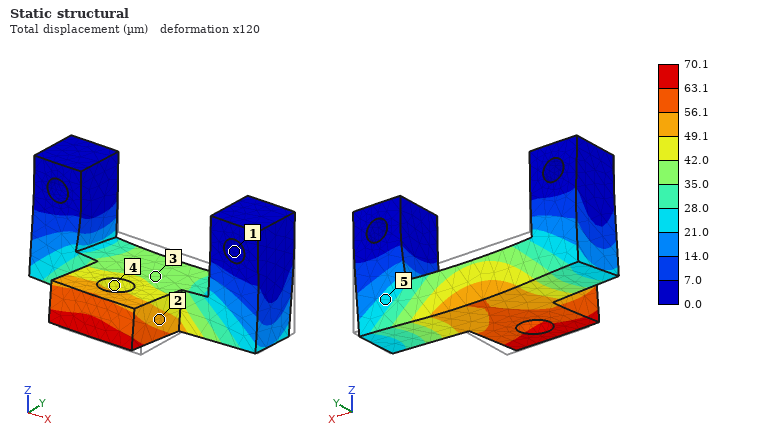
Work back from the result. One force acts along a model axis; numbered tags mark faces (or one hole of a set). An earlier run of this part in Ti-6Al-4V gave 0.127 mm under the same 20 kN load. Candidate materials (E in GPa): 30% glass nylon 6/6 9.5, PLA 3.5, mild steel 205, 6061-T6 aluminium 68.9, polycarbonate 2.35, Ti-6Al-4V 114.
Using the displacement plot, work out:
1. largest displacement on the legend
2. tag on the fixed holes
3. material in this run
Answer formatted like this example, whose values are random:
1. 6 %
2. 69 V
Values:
1. 70.1 µm
2. 1
3. mild steel
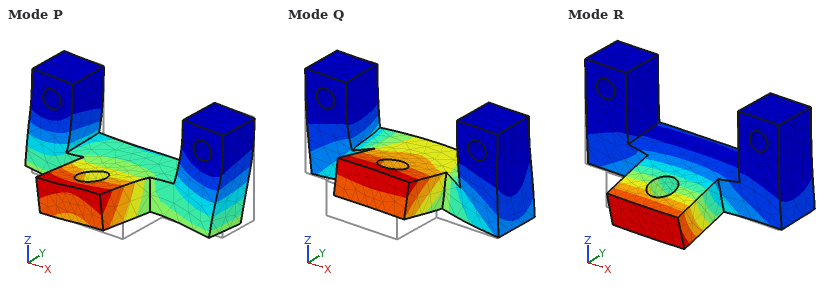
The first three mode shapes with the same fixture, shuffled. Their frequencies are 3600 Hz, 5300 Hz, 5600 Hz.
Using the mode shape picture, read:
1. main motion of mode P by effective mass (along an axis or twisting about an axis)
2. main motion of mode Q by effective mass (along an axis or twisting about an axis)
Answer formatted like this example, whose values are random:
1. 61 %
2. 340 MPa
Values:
1. along X
2. along Y
